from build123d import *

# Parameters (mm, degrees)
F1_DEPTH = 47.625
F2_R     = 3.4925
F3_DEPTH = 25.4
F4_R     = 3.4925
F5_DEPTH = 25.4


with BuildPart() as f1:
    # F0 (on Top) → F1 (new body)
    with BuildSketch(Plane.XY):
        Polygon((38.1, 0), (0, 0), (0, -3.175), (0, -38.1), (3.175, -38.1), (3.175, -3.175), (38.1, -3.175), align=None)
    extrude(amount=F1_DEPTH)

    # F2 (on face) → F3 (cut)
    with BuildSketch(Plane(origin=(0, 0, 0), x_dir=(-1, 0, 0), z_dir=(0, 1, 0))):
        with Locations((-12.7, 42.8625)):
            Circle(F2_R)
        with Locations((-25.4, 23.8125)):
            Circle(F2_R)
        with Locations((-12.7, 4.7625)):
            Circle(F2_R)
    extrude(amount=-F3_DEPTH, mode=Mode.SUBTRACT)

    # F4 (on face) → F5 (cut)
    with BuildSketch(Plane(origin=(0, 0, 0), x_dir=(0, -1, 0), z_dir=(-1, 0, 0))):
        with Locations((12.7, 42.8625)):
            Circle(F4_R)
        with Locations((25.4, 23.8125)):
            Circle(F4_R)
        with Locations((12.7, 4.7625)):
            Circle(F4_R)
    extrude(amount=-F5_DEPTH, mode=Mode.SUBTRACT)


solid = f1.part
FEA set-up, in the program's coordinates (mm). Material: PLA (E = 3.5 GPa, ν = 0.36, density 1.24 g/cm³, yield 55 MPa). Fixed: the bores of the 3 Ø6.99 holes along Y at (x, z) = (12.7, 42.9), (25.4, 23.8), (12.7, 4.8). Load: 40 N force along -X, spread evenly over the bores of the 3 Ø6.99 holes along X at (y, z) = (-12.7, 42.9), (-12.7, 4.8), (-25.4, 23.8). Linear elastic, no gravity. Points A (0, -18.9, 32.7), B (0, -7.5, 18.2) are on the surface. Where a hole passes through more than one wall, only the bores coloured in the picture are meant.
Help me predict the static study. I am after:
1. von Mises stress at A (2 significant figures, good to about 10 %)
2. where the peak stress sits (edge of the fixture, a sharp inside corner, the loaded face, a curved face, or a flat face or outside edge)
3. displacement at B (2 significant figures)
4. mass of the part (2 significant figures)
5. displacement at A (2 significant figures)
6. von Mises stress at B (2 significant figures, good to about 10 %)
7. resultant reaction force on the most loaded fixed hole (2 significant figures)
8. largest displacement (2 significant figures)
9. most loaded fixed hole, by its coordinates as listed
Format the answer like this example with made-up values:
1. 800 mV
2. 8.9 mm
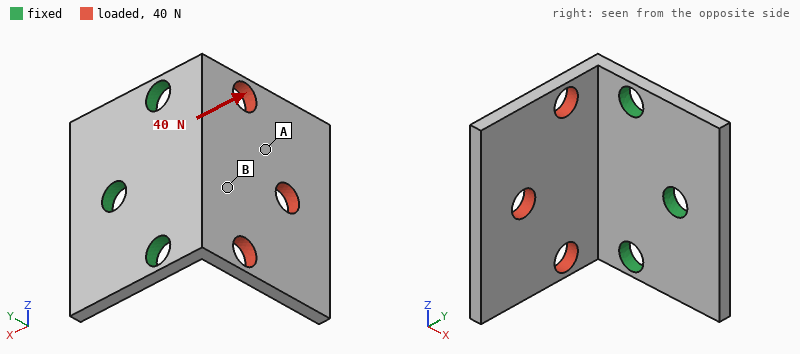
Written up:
1. 1.3 MPa
2. a flat face or outside edge
3. 0.12 mm
4. 13 g
5. 0.33 mm
6. 4.7 MPa
7. 20 N
8. 0.76 mm
9. (25.4, 23.8)
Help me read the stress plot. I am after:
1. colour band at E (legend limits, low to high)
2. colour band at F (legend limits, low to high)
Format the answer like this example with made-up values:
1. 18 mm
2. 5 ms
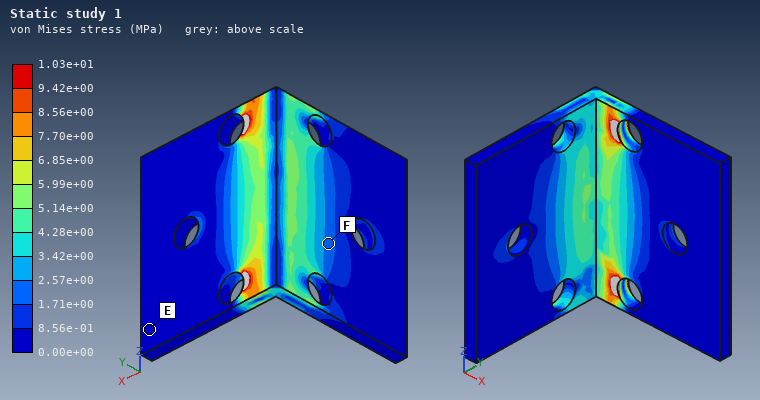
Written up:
1. 0.00e+00 to 8.56e-01 MPa
2. 1.71e+00 to 2.57e+00 MPa
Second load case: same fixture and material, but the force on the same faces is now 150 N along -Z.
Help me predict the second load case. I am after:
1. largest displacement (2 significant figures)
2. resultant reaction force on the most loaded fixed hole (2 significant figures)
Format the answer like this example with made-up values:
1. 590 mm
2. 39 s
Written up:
1. 0.24 mm
2. 100 N
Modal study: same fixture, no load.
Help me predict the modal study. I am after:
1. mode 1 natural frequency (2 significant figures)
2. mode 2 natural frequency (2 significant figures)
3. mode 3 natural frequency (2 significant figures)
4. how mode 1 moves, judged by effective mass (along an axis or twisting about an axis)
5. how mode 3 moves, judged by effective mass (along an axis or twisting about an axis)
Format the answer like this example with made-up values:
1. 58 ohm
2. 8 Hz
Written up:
1. 470 Hz
2. 1100 Hz
3. 1900 Hz
4. along X
5. along Z
